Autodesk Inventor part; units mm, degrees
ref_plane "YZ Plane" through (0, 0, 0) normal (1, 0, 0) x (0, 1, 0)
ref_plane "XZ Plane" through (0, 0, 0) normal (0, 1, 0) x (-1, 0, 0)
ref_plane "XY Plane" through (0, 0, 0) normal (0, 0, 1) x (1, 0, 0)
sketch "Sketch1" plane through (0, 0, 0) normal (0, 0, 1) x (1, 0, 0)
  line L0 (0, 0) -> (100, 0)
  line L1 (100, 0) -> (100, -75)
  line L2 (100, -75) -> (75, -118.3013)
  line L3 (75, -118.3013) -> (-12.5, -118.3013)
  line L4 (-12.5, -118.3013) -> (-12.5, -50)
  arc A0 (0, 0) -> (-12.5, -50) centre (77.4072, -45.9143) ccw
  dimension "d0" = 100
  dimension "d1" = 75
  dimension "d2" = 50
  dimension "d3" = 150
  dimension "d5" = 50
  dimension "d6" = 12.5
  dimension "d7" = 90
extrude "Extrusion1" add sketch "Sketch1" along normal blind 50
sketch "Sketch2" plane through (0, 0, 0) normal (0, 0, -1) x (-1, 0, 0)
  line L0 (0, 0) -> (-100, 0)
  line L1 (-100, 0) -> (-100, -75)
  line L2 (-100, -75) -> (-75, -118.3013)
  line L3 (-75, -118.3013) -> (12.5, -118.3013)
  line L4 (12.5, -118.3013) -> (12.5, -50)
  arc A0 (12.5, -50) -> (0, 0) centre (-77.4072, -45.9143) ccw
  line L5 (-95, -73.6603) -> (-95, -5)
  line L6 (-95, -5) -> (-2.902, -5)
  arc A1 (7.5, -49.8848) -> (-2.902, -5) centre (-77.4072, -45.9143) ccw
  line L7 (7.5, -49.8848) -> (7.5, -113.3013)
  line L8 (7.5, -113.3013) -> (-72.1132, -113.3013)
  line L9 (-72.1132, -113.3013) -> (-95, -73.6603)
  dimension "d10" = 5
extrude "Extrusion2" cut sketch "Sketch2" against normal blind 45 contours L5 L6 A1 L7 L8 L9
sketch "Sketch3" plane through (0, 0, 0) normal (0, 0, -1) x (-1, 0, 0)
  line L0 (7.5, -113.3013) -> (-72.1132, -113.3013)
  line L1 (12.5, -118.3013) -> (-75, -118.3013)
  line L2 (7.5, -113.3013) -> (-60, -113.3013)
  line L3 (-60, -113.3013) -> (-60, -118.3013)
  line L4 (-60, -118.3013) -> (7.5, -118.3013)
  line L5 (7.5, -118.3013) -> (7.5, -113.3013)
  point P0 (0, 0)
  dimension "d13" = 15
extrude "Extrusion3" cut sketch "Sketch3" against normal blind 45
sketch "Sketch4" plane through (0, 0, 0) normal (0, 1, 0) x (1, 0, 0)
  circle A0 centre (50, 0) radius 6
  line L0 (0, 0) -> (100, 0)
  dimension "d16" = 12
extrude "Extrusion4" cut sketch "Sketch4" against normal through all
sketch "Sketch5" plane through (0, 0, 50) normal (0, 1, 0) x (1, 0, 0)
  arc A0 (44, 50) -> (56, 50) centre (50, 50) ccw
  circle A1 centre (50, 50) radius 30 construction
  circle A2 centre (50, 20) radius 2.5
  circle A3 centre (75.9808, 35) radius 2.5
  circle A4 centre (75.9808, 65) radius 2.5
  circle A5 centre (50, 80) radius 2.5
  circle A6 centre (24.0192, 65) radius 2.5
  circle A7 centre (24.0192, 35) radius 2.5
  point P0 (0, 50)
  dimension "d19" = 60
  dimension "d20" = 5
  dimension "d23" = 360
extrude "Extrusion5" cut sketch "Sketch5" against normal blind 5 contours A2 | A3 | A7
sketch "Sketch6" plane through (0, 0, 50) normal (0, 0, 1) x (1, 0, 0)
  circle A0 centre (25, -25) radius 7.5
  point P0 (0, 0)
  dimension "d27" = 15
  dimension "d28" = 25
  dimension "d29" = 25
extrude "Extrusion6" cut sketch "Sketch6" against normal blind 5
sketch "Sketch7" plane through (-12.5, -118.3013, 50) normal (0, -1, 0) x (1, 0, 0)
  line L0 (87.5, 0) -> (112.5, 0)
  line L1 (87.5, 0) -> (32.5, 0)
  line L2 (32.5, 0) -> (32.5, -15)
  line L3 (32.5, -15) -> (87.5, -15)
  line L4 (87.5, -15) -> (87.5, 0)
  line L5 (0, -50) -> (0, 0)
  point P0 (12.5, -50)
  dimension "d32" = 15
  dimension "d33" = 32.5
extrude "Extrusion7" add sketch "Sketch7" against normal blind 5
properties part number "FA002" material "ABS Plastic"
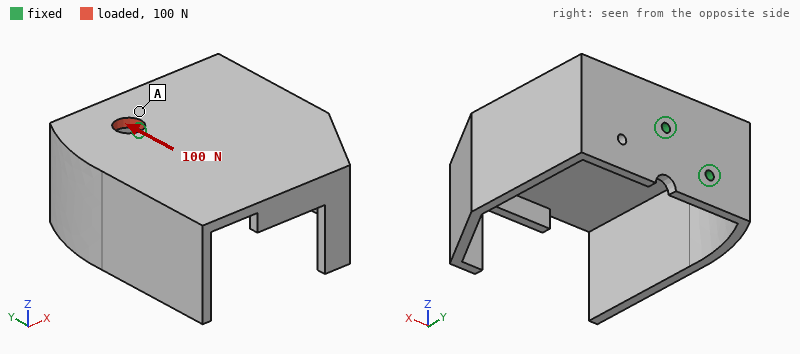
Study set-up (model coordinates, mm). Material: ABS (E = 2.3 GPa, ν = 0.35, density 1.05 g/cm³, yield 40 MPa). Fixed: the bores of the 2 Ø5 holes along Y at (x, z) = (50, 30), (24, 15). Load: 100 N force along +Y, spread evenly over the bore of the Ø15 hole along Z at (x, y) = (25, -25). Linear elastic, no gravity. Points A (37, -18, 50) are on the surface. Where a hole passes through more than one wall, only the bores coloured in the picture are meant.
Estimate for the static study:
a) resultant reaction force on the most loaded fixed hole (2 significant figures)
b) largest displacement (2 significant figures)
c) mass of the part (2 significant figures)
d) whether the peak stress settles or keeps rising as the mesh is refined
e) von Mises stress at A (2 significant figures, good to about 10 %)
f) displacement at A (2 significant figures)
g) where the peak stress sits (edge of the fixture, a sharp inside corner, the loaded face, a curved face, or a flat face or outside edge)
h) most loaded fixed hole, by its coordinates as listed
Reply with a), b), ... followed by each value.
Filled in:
a) 57 N
b) 1.8 mm
c) 150 g
d) keeps rising
e) 0.86 MPa
f) 0.38 mm
g) edge of the fixture
h) (50, 30)
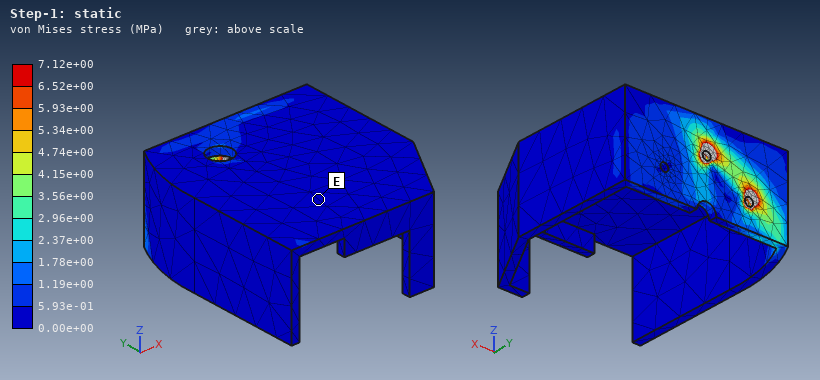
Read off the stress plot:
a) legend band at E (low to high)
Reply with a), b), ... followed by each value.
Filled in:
a) 0.00e+00 to 5.93e-01 MPa
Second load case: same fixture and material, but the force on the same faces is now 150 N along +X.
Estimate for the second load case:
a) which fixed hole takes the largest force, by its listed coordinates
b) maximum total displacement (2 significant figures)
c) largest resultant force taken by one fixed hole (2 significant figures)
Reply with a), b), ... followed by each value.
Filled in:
a) (50, 30)
b) 1.7 mm
c) 190 N
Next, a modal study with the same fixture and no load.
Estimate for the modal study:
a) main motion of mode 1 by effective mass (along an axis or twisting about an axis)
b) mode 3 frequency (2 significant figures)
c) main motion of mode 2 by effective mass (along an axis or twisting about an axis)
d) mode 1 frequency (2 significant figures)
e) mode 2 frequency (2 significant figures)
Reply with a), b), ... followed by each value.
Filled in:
a) along Z
b) 230 Hz
c) along X
d) 74 Hz
e) 100 Hz
